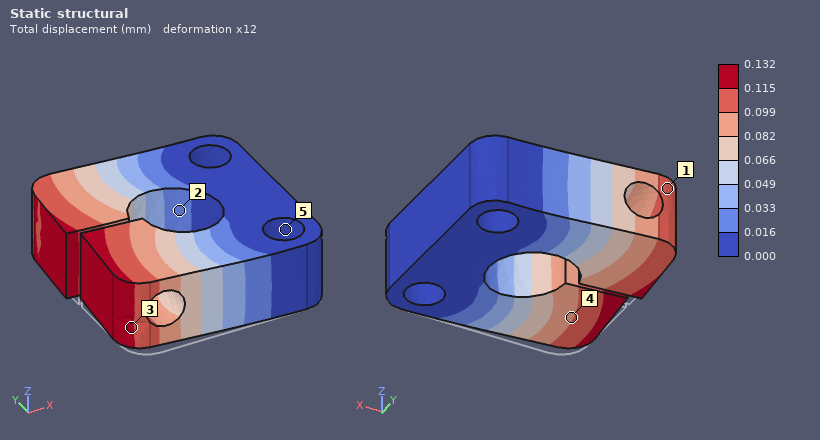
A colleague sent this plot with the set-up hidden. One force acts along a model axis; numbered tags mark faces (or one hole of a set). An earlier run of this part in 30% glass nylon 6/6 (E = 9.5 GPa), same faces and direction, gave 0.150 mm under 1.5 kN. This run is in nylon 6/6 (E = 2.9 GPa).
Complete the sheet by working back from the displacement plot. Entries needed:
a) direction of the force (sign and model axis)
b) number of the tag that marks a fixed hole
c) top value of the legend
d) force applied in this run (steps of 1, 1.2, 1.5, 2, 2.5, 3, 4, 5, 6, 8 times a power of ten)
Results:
+Y
5
0.132 mm
400 N
